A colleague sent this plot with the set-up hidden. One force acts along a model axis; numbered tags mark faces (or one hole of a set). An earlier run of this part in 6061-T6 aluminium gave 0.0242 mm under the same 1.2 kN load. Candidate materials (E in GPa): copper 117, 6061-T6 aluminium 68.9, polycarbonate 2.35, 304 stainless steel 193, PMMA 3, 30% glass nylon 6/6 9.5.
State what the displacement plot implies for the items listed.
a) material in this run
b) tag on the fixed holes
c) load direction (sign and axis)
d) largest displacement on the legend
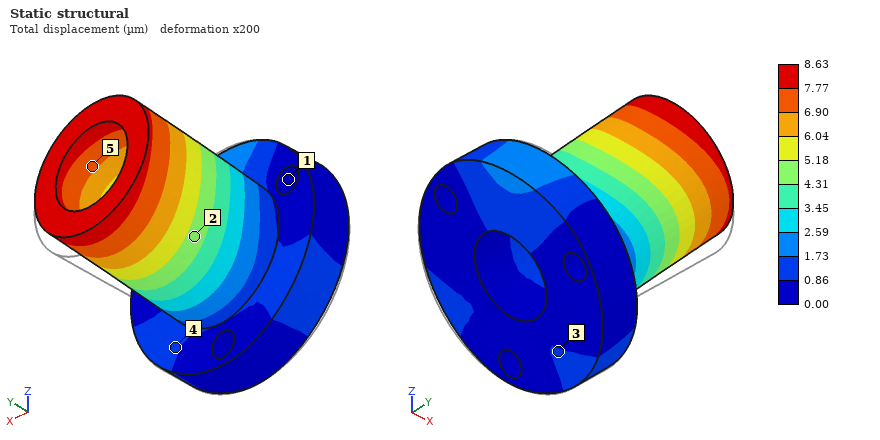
304 stainless steel
1
+Z
8.63 µm
